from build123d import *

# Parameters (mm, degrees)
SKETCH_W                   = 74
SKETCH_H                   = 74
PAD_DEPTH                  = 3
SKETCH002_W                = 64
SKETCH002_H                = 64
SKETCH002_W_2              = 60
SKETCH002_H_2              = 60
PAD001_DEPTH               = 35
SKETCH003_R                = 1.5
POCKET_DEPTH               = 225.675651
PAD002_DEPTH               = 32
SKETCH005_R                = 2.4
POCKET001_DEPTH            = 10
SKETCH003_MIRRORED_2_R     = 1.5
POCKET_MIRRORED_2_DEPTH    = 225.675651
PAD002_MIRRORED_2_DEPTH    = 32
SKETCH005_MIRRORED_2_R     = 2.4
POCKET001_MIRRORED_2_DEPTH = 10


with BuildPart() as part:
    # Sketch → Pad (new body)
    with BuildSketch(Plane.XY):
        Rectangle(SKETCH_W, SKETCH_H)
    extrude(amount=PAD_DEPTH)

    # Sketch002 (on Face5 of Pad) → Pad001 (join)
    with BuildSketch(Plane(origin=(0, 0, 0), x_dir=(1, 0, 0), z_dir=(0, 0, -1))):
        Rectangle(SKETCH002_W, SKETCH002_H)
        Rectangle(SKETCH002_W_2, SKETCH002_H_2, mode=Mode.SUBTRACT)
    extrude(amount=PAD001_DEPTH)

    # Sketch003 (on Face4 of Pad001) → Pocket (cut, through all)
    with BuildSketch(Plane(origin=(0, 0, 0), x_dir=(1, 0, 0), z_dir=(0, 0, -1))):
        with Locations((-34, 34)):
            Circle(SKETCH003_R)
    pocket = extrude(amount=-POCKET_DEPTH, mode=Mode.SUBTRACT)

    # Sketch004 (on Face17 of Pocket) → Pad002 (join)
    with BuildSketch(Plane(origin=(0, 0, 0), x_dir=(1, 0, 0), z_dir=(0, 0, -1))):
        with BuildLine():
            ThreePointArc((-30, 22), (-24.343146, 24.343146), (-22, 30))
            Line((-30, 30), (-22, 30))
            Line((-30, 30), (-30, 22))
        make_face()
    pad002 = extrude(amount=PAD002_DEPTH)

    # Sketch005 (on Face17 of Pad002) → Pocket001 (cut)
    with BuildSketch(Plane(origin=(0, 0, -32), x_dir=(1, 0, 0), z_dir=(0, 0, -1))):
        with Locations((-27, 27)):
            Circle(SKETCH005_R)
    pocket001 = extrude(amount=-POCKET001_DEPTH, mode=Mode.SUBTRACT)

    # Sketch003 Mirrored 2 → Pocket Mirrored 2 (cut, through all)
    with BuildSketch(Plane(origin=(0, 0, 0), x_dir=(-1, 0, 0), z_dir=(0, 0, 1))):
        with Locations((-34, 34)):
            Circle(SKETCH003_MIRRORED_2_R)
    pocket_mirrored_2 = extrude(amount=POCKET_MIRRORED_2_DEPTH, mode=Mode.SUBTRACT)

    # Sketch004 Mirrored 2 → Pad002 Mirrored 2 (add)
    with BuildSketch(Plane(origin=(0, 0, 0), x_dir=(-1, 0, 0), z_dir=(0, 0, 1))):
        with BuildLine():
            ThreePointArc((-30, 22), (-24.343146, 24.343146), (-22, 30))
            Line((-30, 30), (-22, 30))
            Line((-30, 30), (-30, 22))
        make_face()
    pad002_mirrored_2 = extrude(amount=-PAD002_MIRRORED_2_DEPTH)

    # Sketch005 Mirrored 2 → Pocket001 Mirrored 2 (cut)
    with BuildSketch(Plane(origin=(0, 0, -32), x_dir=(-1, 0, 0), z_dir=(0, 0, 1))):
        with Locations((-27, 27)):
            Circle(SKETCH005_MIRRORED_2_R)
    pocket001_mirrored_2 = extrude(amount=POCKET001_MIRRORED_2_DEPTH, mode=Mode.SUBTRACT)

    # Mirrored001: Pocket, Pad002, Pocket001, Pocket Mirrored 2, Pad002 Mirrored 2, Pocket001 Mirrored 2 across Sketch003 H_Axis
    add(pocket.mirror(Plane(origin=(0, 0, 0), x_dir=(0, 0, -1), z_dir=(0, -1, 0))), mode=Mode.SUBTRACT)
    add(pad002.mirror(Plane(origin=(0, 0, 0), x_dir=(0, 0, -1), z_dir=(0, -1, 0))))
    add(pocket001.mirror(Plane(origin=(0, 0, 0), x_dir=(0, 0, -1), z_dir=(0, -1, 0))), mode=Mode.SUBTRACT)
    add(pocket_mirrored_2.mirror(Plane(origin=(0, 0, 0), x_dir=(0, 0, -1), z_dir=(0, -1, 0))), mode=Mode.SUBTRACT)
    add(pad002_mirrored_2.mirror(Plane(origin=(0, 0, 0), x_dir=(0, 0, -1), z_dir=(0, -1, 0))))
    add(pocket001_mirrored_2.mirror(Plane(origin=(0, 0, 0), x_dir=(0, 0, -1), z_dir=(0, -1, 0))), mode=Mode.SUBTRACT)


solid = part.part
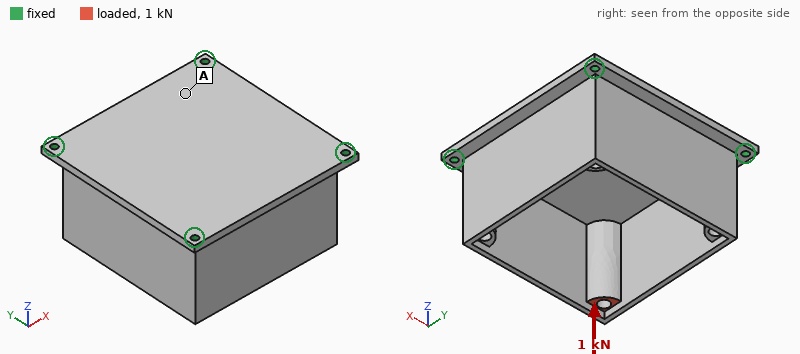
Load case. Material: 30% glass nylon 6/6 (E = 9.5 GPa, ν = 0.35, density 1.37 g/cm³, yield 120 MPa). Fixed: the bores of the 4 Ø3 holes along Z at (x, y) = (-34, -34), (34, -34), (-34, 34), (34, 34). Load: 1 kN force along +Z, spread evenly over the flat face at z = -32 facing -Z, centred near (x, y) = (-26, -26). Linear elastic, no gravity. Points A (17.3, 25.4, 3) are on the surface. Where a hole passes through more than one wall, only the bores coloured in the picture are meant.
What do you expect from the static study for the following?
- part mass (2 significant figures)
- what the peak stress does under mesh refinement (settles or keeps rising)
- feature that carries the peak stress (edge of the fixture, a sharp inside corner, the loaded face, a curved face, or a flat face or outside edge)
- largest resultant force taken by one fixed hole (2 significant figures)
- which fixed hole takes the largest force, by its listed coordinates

54 g
keeps rising
edge of the fixture
850 N
(-34, -34)
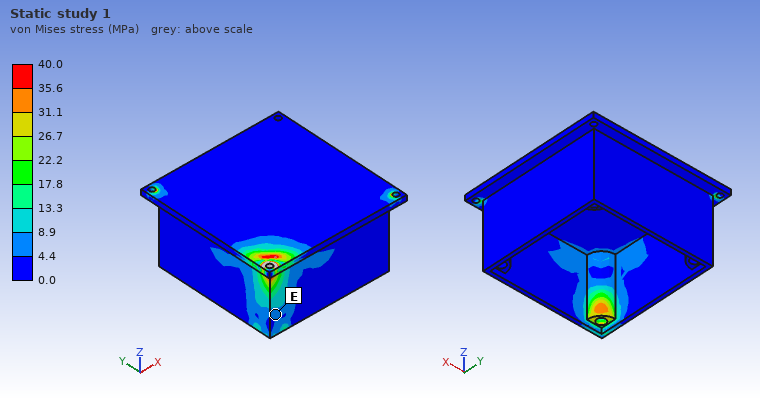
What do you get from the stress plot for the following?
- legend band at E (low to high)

4.4 to 8.9 MPa
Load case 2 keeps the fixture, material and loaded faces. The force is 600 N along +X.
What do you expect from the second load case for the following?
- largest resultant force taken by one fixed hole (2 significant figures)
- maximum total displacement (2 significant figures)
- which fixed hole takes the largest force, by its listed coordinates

450 N
0.38 mm
(34, -34)
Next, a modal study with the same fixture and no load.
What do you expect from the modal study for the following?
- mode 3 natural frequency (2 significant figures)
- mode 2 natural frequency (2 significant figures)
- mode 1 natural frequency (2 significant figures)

2300 Hz
2300 Hz
2100 Hz
